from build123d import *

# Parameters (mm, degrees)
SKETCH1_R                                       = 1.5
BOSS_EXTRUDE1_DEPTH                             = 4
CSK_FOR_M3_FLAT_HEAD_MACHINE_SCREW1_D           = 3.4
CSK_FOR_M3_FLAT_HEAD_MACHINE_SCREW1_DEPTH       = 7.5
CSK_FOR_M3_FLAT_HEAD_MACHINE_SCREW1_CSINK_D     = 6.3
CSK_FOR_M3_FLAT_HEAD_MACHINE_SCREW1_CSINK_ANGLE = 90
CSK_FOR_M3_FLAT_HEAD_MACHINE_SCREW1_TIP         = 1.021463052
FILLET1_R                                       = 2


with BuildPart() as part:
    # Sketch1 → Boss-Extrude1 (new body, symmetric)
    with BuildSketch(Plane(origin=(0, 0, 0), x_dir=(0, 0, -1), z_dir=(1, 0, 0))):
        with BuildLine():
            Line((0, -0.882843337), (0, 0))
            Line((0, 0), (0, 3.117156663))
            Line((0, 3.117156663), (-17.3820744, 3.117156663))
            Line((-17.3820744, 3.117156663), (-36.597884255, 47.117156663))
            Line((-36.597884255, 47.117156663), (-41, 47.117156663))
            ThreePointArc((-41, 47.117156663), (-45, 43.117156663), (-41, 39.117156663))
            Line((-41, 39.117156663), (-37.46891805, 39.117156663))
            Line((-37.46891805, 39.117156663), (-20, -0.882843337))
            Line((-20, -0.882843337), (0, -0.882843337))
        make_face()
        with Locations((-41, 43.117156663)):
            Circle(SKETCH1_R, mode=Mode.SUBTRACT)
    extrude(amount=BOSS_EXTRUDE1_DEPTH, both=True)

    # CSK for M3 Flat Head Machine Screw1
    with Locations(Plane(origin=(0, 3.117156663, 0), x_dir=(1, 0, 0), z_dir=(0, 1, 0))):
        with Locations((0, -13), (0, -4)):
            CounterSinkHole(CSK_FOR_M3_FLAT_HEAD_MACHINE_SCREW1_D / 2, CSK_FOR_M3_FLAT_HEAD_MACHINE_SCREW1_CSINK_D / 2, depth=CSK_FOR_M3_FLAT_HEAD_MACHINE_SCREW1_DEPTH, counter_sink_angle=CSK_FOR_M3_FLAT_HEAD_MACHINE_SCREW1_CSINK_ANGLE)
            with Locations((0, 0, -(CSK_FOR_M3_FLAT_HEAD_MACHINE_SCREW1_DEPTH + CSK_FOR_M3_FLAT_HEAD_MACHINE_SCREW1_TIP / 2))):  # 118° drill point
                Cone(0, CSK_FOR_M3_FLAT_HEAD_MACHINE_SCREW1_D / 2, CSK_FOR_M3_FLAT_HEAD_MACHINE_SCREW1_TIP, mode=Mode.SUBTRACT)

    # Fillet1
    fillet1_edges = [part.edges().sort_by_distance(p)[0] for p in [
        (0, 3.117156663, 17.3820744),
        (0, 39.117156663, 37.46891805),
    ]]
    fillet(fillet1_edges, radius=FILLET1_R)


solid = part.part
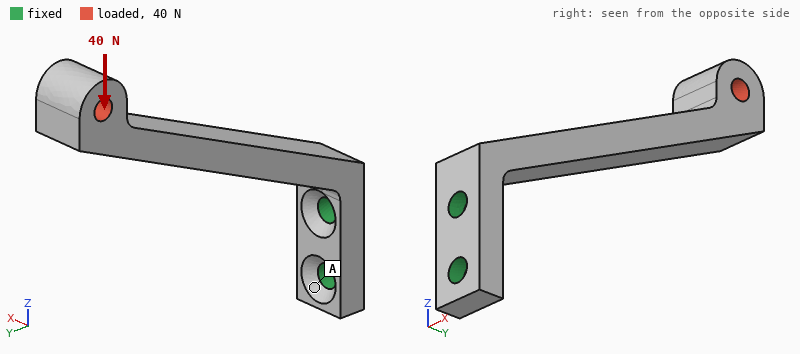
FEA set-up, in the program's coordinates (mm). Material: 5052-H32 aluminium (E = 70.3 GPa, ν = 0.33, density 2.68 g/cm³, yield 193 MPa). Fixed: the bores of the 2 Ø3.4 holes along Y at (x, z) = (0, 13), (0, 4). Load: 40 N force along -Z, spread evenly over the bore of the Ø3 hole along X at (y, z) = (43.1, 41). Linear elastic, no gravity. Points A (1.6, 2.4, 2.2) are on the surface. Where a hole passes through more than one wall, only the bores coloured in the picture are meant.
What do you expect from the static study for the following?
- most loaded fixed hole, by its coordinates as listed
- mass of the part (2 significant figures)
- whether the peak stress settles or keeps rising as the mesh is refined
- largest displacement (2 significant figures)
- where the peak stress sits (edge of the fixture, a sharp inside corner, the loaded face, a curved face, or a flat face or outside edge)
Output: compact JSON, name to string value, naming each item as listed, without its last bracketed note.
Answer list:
{"most loaded fixed hole, by its coordinates as listed": "(0, 4)", "mass of the part": "6.3 g", "whether the peak stress settles or keeps rising as the mesh is refined": "keeps rising", "largest displacement": "0.64 mm", "where the peak stress sits": "edge of the fixture"}
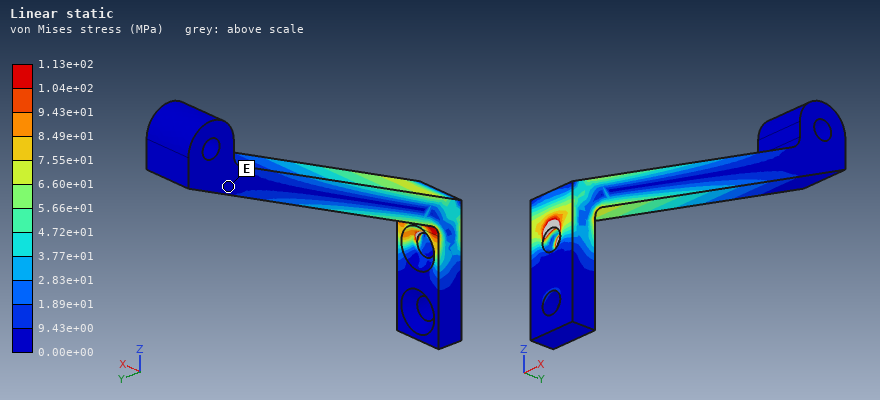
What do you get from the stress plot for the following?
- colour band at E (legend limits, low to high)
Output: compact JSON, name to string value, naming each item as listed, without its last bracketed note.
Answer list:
{"colour band at E": "0.00e+00 to 9.43e+00 MPa"}
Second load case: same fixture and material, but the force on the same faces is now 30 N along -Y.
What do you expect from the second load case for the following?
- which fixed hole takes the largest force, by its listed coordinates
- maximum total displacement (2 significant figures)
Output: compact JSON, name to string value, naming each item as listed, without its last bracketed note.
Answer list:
{"which fixed hole takes the largest force, by its listed coordinates": "(0, 13)", "maximum total displacement": "0.28 mm"}
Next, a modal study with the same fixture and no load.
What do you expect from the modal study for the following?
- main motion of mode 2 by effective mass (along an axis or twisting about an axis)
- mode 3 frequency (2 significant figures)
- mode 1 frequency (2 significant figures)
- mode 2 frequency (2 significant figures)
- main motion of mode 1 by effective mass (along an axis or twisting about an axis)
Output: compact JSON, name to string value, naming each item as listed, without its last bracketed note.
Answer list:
{"main motion of mode 2 by effective mass": "along X", "mode 3 frequency": "5800 Hz", "mode 1 frequency": "870 Hz", "mode 2 frequency": "1400 Hz", "main motion of mode 1 by effective mass": "along Z"}
